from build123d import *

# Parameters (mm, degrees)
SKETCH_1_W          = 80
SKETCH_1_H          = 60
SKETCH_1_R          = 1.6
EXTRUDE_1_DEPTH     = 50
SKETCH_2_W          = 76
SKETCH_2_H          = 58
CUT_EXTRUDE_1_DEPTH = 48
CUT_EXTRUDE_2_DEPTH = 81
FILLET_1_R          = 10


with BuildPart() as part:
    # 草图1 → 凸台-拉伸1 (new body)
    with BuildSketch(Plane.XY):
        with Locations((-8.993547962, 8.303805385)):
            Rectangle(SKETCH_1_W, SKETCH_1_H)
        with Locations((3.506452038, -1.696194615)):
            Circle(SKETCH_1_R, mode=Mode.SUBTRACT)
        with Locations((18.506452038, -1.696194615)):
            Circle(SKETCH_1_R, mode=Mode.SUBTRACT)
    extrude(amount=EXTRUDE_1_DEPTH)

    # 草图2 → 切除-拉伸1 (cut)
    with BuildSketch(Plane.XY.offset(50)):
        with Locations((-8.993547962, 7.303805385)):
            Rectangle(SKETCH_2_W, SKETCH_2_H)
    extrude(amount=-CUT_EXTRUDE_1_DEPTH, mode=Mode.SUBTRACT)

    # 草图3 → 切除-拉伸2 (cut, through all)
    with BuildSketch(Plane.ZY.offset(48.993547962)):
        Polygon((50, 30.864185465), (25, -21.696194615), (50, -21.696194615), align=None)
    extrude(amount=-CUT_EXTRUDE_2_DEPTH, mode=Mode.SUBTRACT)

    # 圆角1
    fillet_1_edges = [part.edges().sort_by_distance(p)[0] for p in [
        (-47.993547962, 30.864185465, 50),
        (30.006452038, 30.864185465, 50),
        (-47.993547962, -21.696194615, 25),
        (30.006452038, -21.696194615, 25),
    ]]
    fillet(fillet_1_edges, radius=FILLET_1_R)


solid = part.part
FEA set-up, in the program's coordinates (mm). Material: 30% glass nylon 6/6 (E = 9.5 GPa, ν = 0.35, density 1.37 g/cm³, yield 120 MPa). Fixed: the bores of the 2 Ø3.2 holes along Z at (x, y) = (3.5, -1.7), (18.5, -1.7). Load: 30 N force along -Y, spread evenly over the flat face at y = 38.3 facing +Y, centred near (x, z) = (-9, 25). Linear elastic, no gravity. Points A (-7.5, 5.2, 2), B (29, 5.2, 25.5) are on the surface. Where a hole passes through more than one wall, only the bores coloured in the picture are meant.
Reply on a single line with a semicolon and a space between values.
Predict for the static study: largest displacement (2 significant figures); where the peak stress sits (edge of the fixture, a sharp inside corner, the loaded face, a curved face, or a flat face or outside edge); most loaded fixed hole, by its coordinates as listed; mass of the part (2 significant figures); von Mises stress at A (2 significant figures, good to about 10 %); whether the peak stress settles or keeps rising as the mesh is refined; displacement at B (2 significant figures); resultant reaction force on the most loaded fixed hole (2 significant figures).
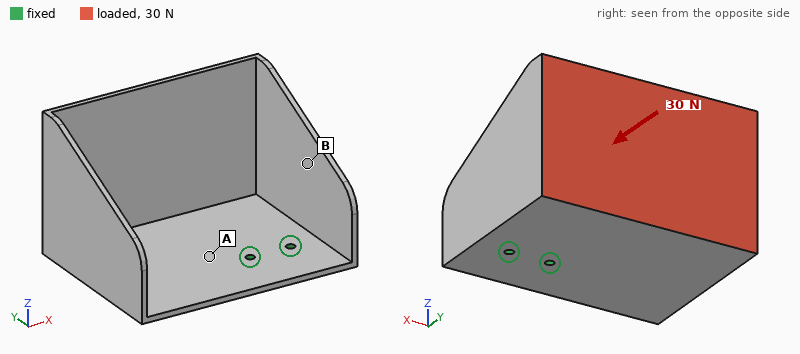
1.3 mm; edge of the fixture; (3.5, -1.7); 35 g; 6.3 MPa; keeps rising; 0.35 mm; 50 N
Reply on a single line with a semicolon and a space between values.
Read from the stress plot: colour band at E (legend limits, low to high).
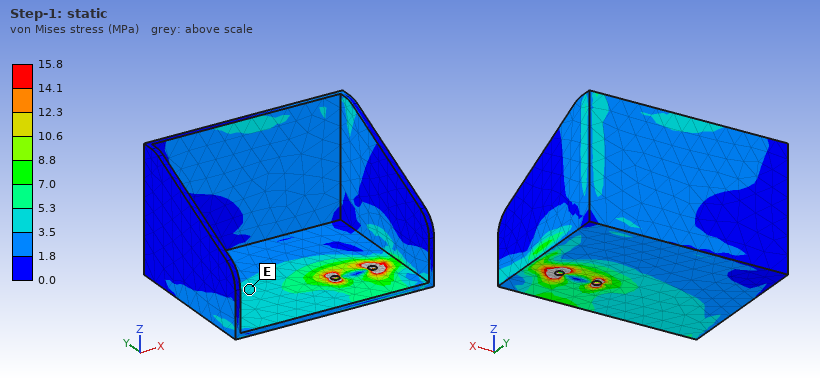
3.5 to 5.3 MPa
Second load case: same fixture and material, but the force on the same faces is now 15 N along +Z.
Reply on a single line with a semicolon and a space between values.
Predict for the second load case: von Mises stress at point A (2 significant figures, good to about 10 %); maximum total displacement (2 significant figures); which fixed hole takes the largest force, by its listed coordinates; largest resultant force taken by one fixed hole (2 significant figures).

6.2 MPa; 1.2 mm; (3.5, -1.7); 19 N
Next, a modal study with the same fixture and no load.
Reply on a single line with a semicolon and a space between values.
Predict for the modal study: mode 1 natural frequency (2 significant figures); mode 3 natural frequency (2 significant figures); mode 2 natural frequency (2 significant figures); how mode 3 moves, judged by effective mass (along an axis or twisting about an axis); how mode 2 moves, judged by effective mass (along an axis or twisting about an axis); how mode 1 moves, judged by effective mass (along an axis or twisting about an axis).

140 Hz; 340 Hz; 190 Hz; along Z; along Y; along Z
